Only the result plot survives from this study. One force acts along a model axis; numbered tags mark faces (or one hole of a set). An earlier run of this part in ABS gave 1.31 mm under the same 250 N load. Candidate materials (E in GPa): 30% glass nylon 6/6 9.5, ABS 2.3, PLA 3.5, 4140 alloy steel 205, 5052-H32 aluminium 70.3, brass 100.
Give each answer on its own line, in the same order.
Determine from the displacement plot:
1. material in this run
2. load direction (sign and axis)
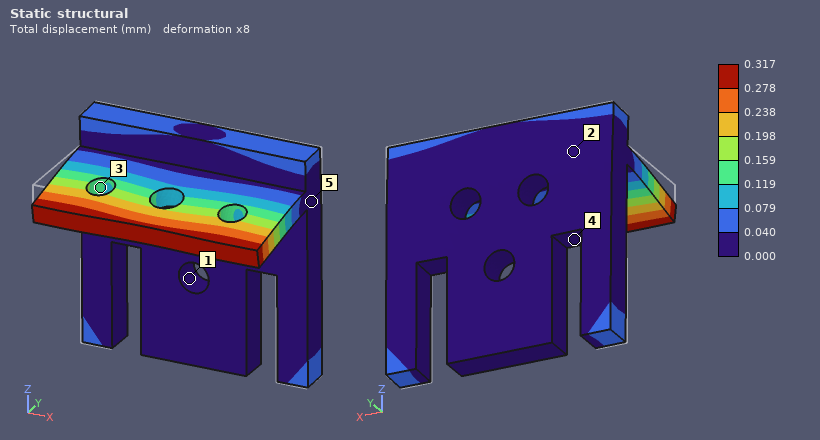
30% glass nylon 6/6
-Z
